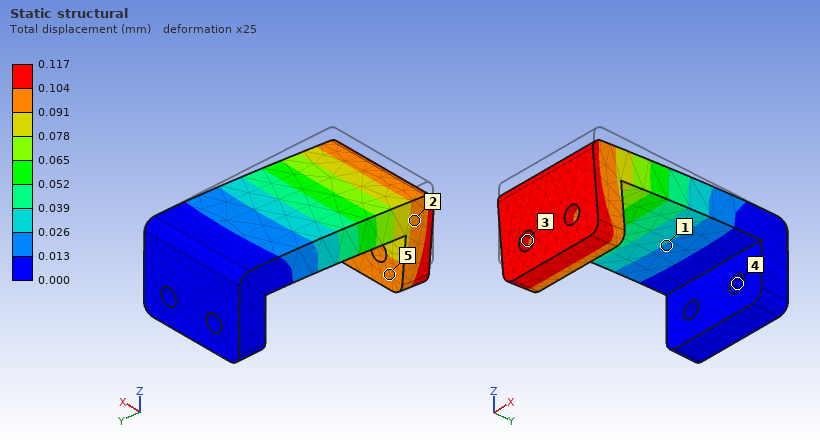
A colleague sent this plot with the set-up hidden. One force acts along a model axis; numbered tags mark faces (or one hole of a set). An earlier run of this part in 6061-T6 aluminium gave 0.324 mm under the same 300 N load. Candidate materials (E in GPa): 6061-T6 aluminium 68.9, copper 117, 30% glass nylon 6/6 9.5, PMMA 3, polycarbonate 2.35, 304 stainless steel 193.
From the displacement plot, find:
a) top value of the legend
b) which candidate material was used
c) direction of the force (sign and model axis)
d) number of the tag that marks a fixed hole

0.117 mm
304 stainless steel
-Z
4
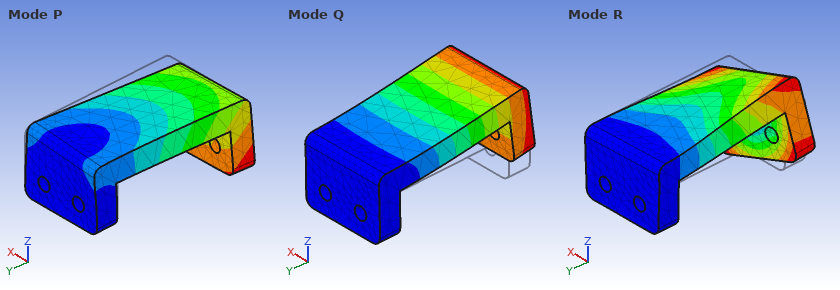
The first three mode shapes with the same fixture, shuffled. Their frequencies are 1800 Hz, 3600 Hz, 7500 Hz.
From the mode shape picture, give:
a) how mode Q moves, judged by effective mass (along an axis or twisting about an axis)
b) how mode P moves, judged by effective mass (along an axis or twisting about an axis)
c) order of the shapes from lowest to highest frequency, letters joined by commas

along Z
along X
Q, P, R
